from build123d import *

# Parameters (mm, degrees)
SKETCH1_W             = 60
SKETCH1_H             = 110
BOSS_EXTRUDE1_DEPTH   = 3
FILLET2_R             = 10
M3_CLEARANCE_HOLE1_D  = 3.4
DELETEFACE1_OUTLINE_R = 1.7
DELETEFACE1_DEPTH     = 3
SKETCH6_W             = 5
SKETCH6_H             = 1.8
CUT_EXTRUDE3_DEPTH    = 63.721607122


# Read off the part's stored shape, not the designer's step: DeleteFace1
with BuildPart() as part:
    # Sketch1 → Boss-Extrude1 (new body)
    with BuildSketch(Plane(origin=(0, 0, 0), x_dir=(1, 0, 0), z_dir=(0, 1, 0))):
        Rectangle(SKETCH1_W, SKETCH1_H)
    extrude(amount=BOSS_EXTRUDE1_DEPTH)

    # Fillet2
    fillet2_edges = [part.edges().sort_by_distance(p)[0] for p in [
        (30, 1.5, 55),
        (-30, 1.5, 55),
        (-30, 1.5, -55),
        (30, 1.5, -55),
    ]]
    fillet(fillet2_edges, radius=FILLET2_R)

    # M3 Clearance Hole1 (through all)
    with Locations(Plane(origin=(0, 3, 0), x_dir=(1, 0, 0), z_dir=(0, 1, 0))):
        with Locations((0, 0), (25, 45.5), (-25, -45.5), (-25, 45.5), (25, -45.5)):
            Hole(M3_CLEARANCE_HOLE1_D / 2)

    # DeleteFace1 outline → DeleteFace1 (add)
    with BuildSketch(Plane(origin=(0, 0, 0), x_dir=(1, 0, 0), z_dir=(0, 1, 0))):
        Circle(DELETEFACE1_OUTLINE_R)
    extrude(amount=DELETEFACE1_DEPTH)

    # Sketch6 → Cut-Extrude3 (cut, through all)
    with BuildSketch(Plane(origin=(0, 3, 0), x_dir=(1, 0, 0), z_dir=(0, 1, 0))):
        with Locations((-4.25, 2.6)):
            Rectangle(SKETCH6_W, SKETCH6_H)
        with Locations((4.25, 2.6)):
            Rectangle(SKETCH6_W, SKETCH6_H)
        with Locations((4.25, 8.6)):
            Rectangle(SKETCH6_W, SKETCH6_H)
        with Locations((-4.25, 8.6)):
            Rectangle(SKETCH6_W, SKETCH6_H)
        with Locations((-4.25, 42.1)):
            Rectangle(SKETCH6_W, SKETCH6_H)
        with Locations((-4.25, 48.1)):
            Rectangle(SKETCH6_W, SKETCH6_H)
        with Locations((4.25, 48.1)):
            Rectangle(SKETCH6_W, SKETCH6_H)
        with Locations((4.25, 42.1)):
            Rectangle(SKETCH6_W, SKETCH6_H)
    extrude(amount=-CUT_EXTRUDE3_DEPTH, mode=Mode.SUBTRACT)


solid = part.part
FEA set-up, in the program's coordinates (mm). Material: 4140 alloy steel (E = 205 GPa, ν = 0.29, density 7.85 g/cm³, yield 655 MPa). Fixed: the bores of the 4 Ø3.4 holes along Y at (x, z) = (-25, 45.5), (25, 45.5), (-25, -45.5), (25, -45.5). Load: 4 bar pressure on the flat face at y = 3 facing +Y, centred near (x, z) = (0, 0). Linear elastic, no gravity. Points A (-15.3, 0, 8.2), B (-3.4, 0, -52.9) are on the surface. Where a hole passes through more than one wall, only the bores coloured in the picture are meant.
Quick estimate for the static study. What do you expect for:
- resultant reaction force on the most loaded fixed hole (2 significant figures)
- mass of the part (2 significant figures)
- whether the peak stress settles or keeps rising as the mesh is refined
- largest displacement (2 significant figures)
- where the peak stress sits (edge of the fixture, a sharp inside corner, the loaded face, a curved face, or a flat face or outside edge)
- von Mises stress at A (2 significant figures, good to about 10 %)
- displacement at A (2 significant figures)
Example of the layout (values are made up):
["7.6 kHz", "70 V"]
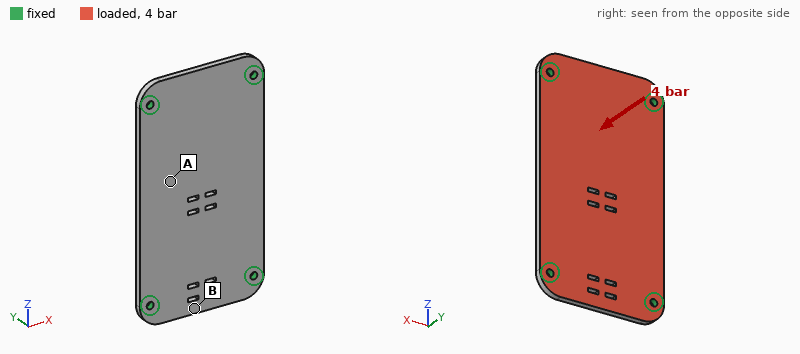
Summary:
["640 N", "150 g", "keeps rising", "0.22 mm", "edge of the fixture", "88 MPa", "0.20 mm"]
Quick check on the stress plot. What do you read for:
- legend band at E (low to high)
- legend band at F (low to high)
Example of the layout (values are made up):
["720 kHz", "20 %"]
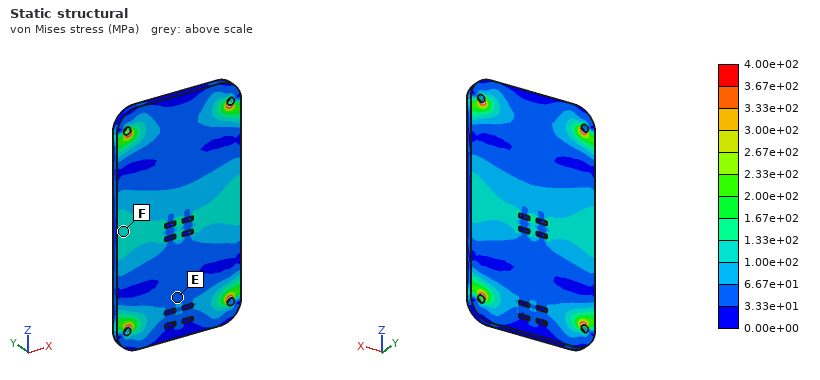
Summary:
["3.33e+01 to 6.67e+01 MPa", "1.00e+02 to 1.33e+02 MPa"]
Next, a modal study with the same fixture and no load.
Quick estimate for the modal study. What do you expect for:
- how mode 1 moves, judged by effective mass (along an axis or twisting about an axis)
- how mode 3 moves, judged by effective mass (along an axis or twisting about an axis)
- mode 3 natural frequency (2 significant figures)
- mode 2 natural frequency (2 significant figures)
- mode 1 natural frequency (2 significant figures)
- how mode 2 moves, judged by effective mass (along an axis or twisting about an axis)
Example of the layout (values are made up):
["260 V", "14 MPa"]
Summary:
["along Y", "twisting about X", "4300 Hz", "2700 Hz", "1600 Hz", "twisting about Z"]
